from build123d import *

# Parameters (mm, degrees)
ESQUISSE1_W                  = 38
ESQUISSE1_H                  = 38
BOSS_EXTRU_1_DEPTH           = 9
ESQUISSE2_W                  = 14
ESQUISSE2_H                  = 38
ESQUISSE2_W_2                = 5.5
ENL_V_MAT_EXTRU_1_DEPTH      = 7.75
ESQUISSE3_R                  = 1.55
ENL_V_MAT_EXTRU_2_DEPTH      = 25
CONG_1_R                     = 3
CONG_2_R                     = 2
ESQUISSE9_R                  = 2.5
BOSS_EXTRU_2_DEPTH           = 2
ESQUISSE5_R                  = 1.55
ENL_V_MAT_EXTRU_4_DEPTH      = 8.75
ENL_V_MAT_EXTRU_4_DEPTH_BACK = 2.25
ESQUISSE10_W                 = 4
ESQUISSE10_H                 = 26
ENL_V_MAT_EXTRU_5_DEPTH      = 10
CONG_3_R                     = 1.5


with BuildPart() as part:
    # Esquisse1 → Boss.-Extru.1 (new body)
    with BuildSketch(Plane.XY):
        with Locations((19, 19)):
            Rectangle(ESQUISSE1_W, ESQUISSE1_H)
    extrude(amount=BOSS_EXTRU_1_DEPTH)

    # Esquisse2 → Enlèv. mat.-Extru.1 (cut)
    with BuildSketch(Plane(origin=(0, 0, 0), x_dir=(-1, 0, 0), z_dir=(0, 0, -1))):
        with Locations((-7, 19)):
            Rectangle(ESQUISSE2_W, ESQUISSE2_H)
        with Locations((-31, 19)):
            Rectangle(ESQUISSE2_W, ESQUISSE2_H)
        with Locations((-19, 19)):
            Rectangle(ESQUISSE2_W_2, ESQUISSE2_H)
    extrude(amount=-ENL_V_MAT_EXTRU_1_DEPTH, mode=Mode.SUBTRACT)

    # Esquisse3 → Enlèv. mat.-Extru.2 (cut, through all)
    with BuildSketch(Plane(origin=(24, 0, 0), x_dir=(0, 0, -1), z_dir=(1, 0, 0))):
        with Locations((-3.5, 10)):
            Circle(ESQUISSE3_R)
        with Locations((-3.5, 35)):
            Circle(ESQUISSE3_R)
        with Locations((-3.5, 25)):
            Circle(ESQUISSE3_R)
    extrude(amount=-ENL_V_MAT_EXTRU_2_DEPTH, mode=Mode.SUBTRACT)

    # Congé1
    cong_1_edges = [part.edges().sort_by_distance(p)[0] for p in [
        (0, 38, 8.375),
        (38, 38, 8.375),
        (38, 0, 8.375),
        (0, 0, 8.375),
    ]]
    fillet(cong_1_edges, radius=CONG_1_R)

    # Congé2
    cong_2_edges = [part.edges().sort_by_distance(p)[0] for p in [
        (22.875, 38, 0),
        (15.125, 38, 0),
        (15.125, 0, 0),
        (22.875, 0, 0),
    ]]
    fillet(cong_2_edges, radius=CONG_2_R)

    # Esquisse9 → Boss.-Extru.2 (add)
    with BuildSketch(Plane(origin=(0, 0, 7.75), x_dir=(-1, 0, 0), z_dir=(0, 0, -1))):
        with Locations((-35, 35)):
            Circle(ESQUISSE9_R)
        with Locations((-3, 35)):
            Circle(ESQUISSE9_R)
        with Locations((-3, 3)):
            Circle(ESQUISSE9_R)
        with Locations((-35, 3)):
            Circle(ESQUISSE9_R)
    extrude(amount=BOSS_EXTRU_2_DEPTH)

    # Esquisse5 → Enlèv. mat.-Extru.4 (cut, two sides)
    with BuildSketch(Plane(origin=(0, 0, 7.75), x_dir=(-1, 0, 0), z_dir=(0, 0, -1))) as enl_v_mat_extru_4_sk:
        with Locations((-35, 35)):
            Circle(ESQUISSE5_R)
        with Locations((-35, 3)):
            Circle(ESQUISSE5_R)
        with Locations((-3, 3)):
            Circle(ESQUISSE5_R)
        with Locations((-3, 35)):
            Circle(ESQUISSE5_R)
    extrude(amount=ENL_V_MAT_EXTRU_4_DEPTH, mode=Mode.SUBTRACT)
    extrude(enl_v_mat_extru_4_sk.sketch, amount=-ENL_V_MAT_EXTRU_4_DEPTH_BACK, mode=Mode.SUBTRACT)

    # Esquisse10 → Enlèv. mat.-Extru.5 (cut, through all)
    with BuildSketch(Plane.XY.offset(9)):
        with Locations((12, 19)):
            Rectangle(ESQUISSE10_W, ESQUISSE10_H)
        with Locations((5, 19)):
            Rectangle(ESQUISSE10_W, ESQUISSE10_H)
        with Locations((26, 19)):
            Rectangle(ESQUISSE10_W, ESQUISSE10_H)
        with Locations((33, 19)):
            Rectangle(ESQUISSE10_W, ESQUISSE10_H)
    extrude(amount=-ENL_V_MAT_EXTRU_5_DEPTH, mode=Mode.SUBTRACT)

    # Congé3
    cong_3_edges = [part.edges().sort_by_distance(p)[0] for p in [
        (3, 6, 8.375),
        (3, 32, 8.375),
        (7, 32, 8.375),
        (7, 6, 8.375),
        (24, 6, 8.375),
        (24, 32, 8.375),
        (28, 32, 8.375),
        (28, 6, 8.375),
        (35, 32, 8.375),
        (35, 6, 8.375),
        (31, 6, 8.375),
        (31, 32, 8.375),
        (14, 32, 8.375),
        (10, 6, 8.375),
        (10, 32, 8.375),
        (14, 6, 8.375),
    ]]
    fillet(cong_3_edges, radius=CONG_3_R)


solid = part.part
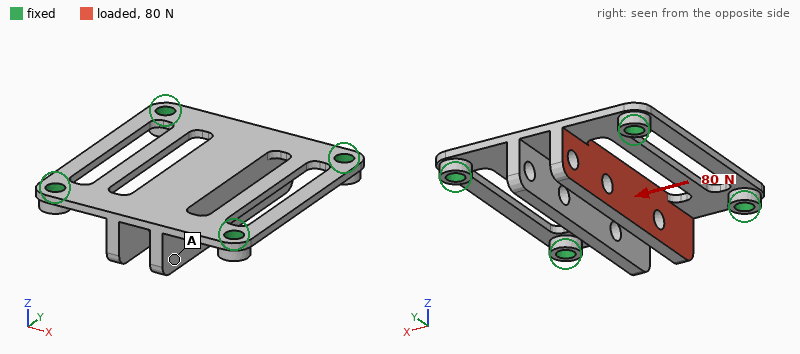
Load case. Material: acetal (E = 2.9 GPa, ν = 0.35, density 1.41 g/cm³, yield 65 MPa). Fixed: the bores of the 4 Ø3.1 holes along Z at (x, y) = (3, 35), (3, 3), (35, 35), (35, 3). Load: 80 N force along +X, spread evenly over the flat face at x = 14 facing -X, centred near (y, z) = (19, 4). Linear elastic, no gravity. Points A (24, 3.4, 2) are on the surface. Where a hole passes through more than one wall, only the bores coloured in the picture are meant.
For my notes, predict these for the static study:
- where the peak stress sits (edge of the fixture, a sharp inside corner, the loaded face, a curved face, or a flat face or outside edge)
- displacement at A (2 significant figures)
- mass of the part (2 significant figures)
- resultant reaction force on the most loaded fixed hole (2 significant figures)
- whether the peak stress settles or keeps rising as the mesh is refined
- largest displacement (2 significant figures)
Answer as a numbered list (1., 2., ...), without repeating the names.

1. a sharp inside corner
2. 0.22 mm
3. 3.6 g
4. 24 N
5. keeps rising
6. 0.55 mm
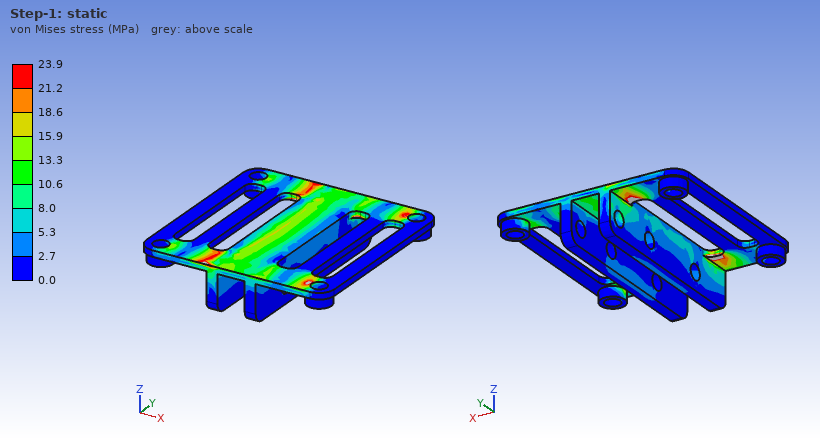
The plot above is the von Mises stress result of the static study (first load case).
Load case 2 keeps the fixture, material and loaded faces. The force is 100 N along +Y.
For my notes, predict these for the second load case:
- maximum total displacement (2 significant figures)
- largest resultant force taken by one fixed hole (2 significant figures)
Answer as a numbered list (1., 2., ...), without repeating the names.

1. 0.36 mm
2. 28 N
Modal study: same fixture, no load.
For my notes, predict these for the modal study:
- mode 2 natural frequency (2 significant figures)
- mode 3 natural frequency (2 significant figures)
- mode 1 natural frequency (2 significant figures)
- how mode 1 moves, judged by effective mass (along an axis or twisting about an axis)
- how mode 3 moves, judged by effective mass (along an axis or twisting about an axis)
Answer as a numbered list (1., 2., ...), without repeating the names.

1. 1500 Hz
2. 1800 Hz
3. 990 Hz
4. along Z
5. along X
